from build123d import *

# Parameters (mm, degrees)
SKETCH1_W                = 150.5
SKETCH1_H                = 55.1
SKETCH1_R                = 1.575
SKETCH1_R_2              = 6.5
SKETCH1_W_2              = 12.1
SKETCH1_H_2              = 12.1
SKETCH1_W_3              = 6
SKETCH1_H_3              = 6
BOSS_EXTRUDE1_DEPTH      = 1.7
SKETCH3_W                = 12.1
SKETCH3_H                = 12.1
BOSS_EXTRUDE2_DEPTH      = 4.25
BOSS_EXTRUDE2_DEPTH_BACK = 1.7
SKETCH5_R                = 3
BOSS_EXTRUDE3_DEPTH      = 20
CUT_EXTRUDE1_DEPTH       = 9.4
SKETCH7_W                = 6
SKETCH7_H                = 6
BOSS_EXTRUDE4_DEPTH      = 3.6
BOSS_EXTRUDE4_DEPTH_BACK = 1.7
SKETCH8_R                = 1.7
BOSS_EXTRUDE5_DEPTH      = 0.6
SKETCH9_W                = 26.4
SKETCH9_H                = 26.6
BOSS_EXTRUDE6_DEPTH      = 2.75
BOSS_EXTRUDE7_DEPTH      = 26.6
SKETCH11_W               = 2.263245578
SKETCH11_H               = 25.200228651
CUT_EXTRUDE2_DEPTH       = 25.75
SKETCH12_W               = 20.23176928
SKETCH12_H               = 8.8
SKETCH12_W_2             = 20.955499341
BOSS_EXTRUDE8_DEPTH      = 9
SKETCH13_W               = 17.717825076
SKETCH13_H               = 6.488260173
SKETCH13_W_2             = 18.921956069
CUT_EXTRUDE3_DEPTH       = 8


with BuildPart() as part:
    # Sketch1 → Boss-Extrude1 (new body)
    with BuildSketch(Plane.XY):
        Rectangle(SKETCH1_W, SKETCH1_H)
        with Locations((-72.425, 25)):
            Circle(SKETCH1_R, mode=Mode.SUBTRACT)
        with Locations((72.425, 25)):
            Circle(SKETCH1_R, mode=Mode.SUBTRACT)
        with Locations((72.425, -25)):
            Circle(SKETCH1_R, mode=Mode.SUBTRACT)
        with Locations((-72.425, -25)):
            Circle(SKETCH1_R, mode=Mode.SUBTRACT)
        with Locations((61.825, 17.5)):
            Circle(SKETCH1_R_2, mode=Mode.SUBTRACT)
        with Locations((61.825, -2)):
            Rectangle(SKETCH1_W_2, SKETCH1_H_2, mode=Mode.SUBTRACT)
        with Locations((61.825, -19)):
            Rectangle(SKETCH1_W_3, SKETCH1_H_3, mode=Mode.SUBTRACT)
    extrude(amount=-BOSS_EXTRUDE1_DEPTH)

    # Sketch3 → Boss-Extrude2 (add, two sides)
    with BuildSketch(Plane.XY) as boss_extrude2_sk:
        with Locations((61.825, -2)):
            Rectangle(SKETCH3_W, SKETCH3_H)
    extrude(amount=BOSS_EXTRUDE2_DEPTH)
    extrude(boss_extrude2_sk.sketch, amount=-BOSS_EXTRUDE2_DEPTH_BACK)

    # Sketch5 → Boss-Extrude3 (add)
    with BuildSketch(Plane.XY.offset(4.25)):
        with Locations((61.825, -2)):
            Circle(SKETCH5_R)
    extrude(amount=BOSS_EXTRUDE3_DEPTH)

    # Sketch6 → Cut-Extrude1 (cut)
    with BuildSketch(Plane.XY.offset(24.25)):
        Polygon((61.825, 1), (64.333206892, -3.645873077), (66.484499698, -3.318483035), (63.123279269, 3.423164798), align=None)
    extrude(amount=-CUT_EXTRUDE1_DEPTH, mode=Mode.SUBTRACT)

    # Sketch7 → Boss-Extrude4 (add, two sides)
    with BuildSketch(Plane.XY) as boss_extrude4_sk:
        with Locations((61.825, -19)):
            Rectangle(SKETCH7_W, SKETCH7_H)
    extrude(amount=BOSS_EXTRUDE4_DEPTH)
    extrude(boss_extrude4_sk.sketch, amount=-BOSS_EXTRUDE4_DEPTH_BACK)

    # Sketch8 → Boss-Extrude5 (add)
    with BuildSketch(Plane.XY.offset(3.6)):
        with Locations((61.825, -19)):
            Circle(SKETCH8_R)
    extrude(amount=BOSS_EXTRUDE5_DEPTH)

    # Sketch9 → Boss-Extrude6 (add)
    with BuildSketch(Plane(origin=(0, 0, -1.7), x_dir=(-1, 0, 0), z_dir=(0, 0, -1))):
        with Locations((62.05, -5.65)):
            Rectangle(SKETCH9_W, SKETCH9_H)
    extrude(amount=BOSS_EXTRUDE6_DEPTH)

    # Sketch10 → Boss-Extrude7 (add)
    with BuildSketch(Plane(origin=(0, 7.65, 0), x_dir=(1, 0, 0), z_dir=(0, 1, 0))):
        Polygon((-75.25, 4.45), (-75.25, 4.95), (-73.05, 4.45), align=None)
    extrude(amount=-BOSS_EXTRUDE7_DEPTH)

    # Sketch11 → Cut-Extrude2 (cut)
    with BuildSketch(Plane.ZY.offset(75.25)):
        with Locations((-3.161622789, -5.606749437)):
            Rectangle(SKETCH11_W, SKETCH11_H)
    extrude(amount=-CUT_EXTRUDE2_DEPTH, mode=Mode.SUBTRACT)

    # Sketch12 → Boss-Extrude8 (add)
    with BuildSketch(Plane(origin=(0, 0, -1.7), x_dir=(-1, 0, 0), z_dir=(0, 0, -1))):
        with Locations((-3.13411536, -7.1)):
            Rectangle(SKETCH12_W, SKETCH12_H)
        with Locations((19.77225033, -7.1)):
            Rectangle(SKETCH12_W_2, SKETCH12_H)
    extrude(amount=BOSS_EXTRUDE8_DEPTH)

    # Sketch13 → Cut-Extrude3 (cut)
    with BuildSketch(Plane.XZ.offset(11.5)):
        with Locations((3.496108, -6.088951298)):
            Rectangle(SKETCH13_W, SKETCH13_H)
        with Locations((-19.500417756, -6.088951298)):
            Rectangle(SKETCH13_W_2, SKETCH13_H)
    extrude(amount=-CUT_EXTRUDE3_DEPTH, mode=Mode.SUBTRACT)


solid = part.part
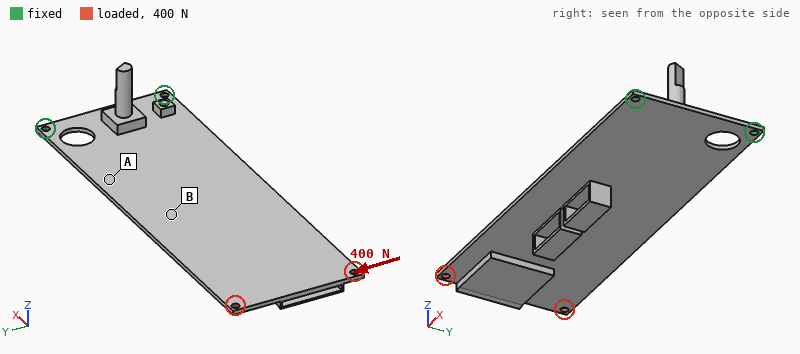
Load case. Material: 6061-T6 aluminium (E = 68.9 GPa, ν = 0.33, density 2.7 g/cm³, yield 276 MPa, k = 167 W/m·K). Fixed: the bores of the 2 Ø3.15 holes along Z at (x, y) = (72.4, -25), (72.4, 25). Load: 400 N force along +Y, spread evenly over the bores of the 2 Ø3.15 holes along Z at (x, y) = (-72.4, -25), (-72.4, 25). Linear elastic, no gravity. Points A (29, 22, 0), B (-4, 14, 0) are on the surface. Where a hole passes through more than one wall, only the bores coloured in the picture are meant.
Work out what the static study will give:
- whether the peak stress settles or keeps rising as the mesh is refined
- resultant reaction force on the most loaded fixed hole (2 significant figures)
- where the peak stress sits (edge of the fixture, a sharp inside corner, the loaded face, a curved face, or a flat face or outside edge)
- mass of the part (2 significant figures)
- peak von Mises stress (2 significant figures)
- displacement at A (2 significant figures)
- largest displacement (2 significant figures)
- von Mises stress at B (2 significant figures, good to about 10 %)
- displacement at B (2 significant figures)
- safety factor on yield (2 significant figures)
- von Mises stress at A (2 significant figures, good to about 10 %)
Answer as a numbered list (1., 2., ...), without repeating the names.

1. settles
2. 1.2 kN
3. a curved face
4. 46 g
5. 270 MPa
6. 0.080 mm
7. 0.38 mm
8. 18 MPa
9. 0.15 mm
10. 1.0
11. 39 MPa
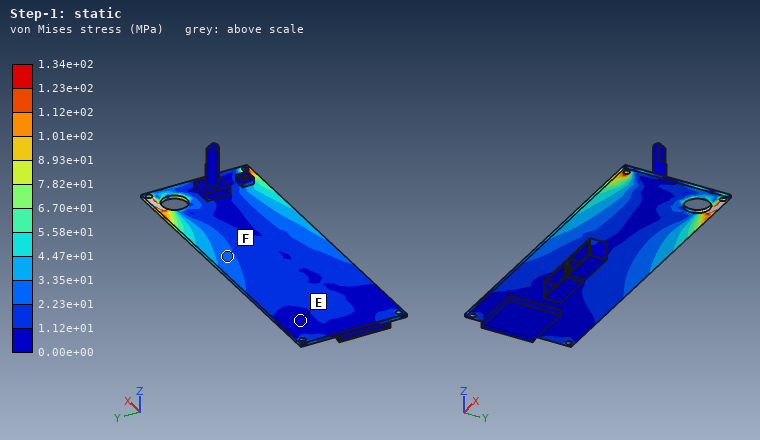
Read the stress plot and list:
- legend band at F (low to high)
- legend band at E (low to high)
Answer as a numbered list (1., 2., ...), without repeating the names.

1. 2.23e+01 to 3.35e+01 MPa
2. 0.00e+00 to 1.12e+01 MPa
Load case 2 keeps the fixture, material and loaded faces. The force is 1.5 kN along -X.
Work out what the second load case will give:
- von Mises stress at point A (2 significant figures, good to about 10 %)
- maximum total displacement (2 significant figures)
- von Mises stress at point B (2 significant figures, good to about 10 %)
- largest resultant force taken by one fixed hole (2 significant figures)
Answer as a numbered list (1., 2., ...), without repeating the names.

1. 18 MPa
2. 0.11 mm
3. 17 MPa
4. 790 N
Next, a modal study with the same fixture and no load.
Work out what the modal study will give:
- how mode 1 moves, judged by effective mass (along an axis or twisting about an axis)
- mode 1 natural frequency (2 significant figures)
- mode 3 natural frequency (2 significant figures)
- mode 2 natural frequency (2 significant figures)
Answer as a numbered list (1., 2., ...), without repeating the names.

1. along Z
2. 54 Hz
3. 400 Hz
4. 390 Hz
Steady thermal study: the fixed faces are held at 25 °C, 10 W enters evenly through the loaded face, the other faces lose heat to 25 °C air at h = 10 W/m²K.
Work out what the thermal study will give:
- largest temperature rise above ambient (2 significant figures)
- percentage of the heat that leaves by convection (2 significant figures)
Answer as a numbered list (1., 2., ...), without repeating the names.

1. 73 K
2. 60 %
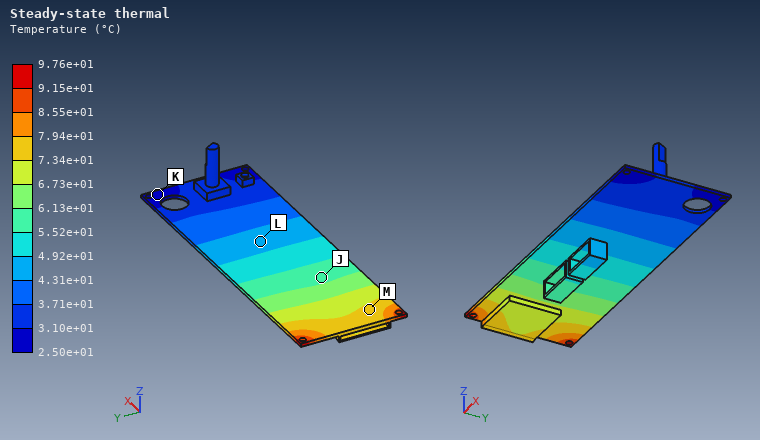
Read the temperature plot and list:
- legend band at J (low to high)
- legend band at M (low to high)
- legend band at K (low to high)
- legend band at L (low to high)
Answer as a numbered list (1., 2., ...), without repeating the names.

1. 5.52e+01 to 6.13e+01 °C
2. 7.34e+01 to 7.94e+01 °C
3. 2.50e+01 to 3.10e+01 °C
4. 4.31e+01 to 4.92e+01 °C
